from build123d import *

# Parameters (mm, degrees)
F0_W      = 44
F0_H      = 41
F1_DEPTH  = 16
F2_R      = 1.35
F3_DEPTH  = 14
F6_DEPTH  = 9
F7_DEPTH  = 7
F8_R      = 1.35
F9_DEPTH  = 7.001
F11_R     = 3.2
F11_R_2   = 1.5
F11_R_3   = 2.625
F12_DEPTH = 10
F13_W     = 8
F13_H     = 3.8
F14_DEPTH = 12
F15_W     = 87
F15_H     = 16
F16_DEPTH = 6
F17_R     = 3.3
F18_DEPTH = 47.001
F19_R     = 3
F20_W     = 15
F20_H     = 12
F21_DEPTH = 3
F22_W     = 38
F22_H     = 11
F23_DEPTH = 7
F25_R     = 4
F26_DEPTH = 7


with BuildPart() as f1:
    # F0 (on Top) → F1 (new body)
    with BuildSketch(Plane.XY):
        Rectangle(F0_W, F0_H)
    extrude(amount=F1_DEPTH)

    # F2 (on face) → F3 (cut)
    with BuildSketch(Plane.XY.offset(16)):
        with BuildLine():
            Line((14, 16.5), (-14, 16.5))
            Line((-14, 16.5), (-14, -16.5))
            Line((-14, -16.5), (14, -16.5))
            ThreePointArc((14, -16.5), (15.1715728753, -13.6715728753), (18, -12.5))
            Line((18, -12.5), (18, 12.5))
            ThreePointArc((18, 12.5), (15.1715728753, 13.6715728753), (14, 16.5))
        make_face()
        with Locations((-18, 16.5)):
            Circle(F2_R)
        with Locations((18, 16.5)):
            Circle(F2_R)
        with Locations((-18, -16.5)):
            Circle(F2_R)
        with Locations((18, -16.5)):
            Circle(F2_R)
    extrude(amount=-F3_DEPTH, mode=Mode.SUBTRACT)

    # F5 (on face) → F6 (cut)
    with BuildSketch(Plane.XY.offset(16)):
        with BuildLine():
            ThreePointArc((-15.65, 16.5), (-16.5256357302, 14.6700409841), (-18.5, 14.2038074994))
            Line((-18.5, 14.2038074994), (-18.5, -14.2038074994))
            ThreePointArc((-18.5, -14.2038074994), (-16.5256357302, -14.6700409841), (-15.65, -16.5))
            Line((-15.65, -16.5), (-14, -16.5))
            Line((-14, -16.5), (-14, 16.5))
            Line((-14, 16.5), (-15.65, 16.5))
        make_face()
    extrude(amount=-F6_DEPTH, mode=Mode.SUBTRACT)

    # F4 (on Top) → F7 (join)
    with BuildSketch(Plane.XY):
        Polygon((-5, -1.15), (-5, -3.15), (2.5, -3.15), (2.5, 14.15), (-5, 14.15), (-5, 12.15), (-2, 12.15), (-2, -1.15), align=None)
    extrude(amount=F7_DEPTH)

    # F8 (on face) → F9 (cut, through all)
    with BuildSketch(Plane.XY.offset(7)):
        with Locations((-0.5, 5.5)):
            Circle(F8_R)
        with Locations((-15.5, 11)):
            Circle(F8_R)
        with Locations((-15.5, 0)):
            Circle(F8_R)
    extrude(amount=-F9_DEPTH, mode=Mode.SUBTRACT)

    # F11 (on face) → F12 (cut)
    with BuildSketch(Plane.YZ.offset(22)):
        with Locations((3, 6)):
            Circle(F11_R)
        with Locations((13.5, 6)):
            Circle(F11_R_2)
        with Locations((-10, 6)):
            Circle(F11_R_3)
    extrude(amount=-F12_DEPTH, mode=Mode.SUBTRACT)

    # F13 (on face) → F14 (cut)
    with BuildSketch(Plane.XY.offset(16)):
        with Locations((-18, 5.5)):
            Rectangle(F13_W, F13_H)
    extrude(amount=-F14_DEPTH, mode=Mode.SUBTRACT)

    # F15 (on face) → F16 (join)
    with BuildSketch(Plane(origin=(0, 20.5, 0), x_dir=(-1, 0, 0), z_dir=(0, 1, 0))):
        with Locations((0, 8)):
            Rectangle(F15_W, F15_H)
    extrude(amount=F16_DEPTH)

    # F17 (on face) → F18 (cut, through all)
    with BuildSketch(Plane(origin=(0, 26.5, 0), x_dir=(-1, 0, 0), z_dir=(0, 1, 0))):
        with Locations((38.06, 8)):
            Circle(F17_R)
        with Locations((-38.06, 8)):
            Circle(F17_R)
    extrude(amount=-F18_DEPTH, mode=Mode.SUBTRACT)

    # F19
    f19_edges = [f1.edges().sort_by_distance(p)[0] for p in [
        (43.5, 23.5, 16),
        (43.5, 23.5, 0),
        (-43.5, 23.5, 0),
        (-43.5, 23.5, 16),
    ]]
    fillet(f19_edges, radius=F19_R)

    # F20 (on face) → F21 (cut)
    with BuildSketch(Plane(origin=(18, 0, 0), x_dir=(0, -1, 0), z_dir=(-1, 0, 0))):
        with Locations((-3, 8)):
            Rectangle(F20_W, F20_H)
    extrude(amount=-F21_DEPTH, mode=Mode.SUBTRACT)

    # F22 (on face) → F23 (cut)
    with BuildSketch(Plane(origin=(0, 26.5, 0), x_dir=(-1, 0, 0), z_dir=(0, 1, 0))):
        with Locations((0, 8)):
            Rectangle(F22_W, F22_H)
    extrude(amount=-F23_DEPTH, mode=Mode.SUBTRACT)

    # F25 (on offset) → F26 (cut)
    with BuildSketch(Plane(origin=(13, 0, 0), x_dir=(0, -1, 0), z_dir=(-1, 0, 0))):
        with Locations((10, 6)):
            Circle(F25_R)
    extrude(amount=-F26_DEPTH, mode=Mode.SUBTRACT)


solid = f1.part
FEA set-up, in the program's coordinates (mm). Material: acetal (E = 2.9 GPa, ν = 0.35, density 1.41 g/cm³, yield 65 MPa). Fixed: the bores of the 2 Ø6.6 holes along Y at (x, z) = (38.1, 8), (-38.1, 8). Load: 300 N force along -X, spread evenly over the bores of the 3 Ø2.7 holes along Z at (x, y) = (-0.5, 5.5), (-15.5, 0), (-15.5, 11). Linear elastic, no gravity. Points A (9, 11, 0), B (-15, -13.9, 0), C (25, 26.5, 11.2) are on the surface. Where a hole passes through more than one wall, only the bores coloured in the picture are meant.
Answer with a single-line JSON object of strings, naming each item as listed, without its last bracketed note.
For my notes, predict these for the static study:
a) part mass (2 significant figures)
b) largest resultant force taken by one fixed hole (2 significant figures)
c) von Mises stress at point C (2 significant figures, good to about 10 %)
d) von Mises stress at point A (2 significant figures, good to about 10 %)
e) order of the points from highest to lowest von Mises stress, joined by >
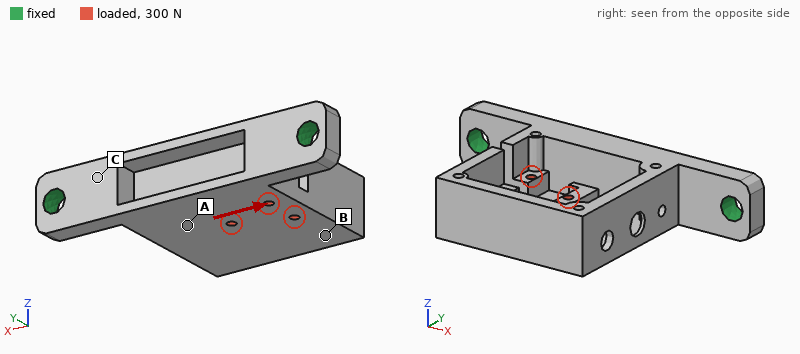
{"part mass": "24 g", "largest resultant force taken by one fixed hole": "180 N", "von Mises stress at point C": "2.5 MPa", "von Mises stress at point A": "4.6 MPa", "order of the points from highest to lowest von Mises stress, joined by >": "A > C > B"}
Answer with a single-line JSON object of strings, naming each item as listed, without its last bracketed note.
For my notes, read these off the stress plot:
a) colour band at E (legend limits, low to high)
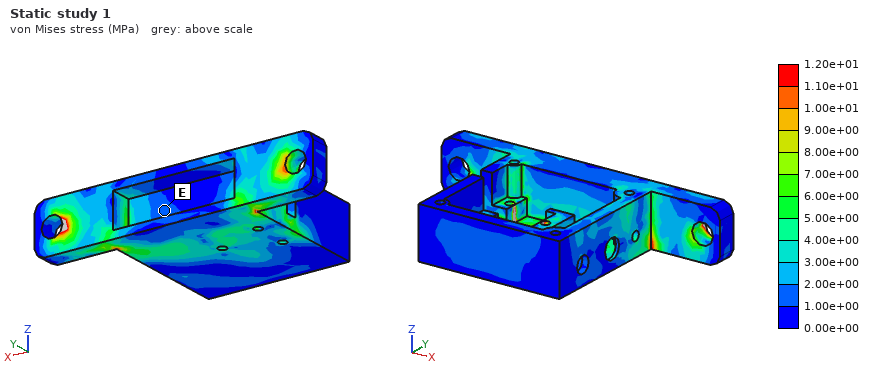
{"colour band at E": "1.00e+00 to 2.00e+00 MPa"}
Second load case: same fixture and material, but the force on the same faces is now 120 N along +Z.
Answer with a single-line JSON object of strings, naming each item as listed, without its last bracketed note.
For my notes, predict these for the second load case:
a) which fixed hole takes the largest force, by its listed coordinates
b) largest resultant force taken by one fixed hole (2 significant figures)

{"which fixed hole takes the largest force, by its listed coordinates": "(-38.1, 8)", "largest resultant force taken by one fixed hole": "79 N"}
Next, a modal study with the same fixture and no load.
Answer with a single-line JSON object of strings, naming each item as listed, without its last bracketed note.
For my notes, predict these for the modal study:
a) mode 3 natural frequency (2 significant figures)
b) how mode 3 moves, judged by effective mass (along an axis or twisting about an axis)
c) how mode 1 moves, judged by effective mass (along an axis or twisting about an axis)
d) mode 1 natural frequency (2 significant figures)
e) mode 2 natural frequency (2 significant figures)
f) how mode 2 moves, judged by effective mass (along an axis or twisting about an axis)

{"mode 3 natural frequency": "1400 Hz", "how mode 3 moves, judged by effective mass": "along Y", "how mode 1 moves, judged by effective mass": "along Z", "mode 1 natural frequency": "400 Hz", "mode 2 natural frequency": "870 Hz", "how mode 2 moves, judged by effective mass": "along X"}
